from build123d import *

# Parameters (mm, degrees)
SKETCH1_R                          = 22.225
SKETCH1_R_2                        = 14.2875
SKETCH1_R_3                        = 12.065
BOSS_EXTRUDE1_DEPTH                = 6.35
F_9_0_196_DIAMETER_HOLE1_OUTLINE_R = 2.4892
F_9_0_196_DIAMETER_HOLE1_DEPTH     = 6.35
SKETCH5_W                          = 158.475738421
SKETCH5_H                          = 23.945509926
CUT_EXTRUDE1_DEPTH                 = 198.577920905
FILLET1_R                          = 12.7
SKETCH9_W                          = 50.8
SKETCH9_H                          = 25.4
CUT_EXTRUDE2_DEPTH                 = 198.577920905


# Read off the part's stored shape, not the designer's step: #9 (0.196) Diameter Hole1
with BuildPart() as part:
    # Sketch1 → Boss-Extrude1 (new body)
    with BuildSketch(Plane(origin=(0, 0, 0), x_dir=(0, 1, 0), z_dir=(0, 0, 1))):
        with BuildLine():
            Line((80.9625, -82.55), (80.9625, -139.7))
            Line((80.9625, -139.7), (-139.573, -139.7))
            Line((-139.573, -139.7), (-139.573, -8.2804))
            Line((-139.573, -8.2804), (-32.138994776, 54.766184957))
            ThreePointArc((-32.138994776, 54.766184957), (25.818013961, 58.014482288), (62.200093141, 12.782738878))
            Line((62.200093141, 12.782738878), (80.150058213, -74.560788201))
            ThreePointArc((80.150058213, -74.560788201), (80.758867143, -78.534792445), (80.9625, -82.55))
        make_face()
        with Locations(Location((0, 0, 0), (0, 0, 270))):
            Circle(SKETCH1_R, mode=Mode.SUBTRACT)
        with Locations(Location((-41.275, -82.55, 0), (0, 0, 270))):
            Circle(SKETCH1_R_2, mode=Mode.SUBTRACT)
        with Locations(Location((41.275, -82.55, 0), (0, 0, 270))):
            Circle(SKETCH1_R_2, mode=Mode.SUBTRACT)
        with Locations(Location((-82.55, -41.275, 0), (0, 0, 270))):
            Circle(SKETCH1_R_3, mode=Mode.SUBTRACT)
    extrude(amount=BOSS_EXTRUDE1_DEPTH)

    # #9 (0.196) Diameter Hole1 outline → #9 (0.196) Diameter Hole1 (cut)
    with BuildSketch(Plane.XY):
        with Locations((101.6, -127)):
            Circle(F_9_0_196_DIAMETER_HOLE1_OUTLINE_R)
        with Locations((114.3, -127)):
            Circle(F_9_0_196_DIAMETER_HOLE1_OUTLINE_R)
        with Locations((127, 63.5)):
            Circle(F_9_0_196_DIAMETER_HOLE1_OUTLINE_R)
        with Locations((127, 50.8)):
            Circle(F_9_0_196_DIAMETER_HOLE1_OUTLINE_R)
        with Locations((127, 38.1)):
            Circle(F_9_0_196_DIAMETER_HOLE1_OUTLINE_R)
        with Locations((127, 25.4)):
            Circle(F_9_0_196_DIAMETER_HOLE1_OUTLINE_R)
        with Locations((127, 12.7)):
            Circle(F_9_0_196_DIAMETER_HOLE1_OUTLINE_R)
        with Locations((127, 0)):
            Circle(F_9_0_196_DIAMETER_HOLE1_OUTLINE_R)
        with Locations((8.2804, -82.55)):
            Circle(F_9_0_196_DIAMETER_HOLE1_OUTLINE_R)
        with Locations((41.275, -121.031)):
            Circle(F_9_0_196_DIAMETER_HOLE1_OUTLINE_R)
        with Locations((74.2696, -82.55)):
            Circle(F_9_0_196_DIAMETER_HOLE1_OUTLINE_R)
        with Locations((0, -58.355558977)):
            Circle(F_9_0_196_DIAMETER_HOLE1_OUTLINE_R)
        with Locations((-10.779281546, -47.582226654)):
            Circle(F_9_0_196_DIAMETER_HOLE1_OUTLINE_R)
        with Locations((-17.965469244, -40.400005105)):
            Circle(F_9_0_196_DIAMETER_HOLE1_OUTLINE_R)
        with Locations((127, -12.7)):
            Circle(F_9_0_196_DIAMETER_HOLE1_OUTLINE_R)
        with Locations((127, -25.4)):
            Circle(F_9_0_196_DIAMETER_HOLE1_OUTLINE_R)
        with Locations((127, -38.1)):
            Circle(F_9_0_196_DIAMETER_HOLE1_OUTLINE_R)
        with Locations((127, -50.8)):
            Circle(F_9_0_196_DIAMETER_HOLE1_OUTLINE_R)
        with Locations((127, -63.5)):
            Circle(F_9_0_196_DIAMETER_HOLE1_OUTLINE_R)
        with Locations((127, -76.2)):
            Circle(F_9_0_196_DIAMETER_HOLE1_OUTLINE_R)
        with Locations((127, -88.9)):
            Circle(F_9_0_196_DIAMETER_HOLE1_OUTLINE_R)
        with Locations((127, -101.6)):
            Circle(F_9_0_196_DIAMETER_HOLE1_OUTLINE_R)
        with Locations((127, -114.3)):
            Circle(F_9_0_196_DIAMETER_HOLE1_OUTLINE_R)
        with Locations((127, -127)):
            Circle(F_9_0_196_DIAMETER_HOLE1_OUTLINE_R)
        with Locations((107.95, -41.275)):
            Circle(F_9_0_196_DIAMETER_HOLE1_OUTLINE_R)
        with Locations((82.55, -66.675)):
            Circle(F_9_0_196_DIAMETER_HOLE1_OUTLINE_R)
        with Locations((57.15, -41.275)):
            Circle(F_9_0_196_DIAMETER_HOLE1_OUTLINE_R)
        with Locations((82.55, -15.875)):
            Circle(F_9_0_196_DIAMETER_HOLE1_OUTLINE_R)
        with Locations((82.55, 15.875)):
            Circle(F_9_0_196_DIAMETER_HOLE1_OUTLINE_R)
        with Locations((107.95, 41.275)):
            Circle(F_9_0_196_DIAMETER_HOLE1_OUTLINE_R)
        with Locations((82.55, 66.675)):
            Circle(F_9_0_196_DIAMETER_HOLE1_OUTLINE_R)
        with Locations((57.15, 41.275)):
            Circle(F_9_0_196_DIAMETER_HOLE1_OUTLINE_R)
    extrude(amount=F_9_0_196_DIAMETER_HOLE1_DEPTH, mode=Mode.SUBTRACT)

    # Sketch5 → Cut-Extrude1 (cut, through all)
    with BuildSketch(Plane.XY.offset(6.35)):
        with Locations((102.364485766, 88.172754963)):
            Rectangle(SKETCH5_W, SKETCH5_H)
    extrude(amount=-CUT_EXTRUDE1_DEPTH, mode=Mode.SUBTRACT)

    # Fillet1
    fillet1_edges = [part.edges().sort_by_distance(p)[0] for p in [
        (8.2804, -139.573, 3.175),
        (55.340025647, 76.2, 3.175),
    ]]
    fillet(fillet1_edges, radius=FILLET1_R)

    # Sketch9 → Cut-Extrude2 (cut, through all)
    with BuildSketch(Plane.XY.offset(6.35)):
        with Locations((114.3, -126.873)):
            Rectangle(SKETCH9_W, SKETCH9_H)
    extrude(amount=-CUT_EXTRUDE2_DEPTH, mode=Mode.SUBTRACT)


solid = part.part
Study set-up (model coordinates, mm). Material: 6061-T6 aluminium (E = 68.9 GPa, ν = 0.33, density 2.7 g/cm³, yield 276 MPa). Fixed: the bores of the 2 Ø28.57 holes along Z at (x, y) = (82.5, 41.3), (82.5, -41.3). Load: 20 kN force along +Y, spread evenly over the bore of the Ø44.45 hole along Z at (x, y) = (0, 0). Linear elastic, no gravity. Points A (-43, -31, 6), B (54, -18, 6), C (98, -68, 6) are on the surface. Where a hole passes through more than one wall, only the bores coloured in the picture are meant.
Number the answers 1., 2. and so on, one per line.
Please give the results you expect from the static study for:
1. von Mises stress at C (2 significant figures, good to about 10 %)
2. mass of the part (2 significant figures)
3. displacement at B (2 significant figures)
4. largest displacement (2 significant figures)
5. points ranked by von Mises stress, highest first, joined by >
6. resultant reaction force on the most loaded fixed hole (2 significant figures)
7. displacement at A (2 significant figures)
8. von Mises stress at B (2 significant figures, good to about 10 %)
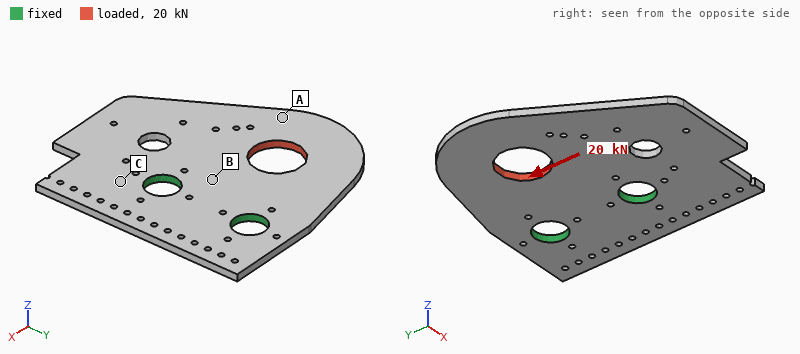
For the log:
1. 24 MPa
2. 550 g
3. 0.025 mm
4. 0.16 mm
5. B > C > A
6. 18 kN
7. 0.15 mm
8. 55 MPa
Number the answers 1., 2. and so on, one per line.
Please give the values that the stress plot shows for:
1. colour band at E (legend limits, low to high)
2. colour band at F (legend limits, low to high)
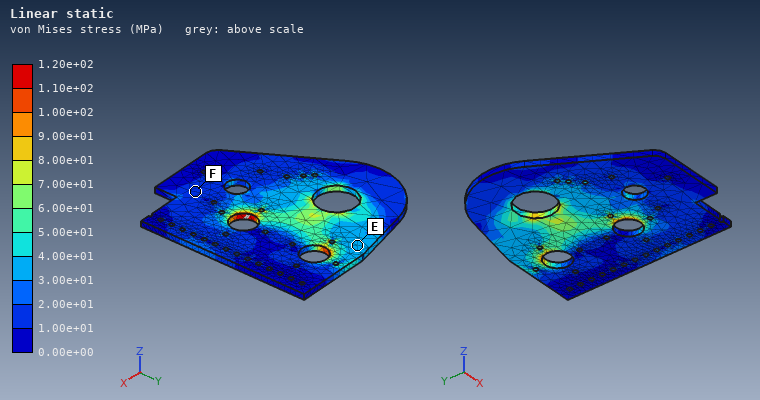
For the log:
1. 3.00e+01 to 4.00e+01 MPa
2. 1.00e+01 to 2.00e+01 MPa
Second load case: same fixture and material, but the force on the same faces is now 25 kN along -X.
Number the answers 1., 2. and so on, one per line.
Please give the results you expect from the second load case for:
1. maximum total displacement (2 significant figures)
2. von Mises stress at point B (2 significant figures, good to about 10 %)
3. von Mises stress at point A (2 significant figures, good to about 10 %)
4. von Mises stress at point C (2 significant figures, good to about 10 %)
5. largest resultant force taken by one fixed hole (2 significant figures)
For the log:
1. 67 µm
2. 28 MPa
3. 18 MPa
4. 7.8 MPa
5. 13 kN
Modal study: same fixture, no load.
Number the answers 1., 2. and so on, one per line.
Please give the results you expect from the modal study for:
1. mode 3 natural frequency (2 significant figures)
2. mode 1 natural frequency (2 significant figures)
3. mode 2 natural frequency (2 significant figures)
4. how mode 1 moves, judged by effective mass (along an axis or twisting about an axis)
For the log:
1. 940 Hz
2. 360 Hz
3. 560 Hz
4. along Z
